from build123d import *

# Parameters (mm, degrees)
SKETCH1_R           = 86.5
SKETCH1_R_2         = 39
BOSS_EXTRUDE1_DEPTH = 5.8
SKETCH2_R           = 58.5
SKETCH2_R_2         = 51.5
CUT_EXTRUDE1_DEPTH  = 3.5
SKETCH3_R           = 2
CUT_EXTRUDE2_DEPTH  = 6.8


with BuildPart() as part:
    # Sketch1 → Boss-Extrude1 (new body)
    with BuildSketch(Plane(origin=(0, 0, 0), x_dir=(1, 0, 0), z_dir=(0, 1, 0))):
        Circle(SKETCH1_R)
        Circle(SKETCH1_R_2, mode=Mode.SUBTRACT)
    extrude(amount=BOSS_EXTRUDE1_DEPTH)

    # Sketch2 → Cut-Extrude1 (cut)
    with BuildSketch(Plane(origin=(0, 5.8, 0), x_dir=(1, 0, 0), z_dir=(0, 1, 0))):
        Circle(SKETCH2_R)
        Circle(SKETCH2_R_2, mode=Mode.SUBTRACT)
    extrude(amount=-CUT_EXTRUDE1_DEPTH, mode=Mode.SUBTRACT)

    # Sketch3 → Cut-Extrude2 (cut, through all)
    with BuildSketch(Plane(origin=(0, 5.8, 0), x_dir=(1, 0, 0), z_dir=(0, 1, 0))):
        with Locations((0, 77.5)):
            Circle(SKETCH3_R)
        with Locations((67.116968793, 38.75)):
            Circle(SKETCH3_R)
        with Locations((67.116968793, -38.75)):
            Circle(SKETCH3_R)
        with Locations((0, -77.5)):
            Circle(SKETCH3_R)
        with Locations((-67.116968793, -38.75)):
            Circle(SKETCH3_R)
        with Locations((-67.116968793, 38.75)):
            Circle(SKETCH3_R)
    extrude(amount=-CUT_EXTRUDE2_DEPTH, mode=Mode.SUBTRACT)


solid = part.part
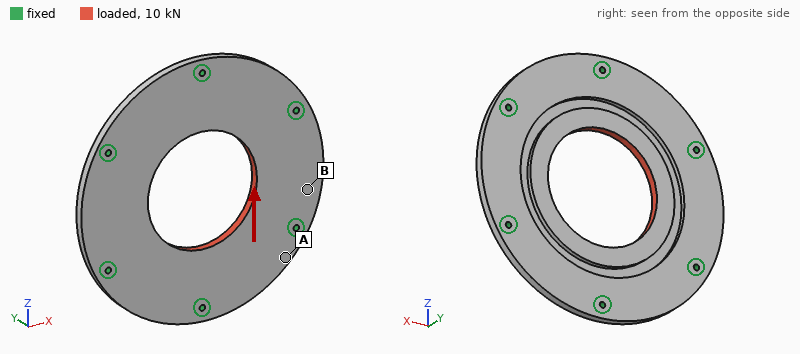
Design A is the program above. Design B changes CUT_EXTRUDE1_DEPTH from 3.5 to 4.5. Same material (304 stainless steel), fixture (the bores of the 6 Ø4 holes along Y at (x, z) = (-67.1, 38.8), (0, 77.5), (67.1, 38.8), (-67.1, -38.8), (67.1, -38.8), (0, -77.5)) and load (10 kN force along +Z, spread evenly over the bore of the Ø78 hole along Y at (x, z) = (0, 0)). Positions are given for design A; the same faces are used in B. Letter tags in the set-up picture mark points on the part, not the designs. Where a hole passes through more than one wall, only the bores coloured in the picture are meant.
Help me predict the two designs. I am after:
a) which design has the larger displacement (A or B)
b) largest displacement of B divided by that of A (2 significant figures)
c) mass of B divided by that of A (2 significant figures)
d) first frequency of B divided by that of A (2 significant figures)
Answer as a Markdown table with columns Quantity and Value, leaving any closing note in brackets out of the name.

| Quantity | Value |
|---|---|
| which design has the larger displacement | B |
| largest displacement of B divided by that of A | 1.7 |
| mass of B divided by that of A | 0.98 |
| first frequency of B divided by that of A | 0.99 |
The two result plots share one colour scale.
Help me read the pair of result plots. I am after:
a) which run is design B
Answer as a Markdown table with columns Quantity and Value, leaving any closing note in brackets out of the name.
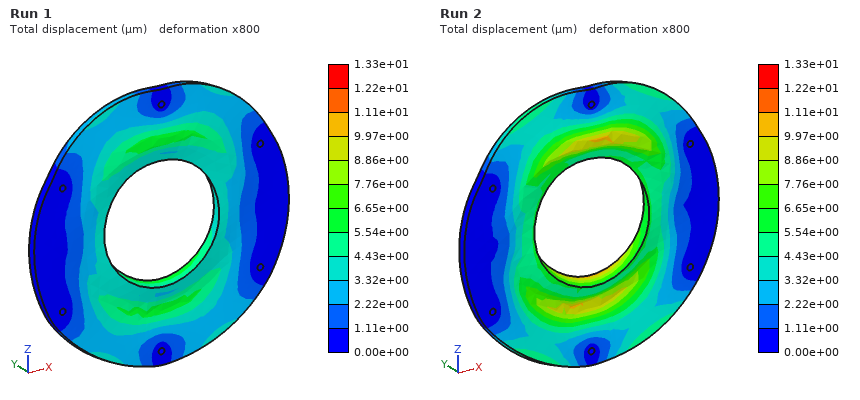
| Quantity | Value |
|---|---|
| which run is design B | Run 2 |
